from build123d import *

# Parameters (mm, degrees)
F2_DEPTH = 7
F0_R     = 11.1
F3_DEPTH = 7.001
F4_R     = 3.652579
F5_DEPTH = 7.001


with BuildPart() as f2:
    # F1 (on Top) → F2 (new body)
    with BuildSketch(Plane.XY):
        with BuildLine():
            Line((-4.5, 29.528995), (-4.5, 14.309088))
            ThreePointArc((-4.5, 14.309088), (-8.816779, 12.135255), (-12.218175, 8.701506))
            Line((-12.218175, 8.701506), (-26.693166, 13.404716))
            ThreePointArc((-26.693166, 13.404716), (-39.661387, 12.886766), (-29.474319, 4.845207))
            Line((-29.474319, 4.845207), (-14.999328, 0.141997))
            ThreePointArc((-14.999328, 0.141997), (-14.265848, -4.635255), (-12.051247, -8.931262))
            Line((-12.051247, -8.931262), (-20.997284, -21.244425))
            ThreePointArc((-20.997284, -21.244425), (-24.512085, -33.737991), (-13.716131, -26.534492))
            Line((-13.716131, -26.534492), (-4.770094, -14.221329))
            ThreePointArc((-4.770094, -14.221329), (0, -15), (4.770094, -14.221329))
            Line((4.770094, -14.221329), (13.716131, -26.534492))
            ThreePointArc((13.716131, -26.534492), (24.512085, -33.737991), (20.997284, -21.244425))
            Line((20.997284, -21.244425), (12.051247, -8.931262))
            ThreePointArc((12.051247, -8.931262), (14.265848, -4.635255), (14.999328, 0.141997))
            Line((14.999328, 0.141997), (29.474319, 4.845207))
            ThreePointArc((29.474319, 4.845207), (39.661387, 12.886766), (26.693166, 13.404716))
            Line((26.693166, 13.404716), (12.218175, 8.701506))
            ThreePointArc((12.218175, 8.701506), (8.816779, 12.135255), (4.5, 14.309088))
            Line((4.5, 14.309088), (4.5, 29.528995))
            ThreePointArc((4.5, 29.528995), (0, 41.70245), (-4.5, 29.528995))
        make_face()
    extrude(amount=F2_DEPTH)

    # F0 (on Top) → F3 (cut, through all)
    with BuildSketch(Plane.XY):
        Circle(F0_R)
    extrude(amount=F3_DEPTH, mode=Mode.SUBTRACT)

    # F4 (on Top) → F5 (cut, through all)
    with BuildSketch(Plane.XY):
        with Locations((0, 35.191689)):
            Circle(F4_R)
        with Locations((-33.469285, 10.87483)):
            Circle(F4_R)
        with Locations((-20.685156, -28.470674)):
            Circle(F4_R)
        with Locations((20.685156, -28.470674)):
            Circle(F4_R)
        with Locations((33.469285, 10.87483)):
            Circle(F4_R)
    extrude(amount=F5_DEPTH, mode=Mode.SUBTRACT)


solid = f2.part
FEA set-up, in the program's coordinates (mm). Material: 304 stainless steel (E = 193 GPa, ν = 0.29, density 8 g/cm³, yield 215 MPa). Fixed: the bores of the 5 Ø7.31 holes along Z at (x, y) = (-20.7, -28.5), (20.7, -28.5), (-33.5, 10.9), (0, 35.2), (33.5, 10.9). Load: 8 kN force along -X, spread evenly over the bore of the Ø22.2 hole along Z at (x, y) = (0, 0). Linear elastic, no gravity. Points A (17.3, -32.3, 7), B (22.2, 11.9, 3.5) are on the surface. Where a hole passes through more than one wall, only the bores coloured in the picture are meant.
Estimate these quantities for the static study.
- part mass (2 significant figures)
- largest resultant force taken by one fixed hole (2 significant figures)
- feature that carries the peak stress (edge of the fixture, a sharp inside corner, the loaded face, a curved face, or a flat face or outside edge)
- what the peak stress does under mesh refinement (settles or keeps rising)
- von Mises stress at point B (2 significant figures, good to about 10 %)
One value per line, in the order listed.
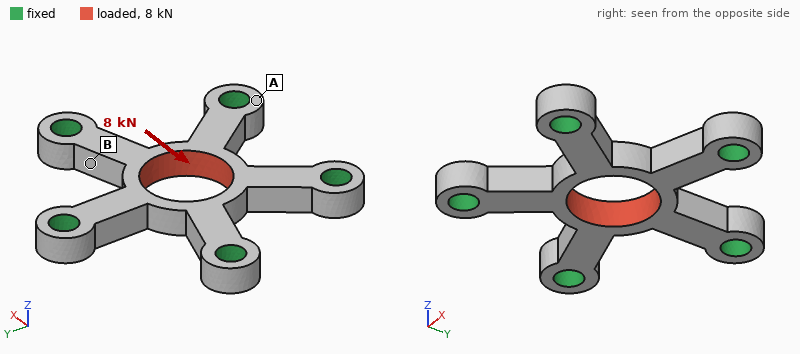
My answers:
83 g
2.7 kN
a sharp inside corner
keeps rising
34 MPa
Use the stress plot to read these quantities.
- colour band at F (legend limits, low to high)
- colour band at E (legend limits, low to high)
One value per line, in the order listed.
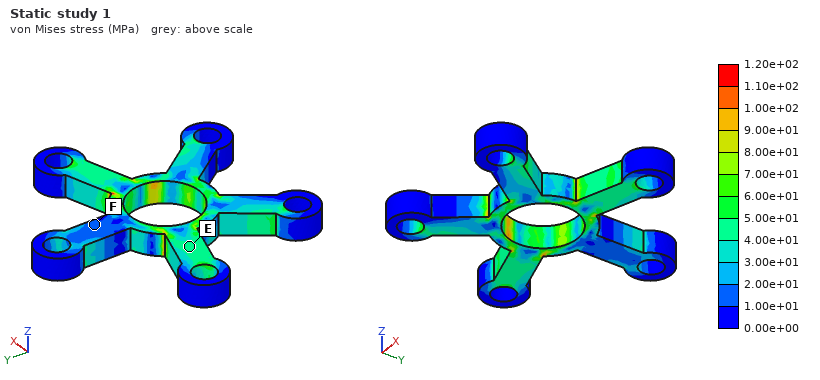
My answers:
1.00e+01 to 2.00e+01 MPa
4.00e+01 to 5.00e+01 MPa
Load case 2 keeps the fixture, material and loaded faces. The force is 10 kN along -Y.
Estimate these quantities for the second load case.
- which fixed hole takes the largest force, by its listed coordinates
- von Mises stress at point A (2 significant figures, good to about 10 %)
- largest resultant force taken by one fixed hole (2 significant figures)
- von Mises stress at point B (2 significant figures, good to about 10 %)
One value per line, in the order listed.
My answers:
(0, 35.2)
12 MPa
3.6 kN
49 MPa
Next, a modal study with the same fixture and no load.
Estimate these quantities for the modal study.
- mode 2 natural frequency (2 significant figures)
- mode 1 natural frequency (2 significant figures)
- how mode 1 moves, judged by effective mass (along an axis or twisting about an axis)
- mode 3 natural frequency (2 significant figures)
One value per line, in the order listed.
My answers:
18 kHz
11 kHz
along Z
18 kHz
